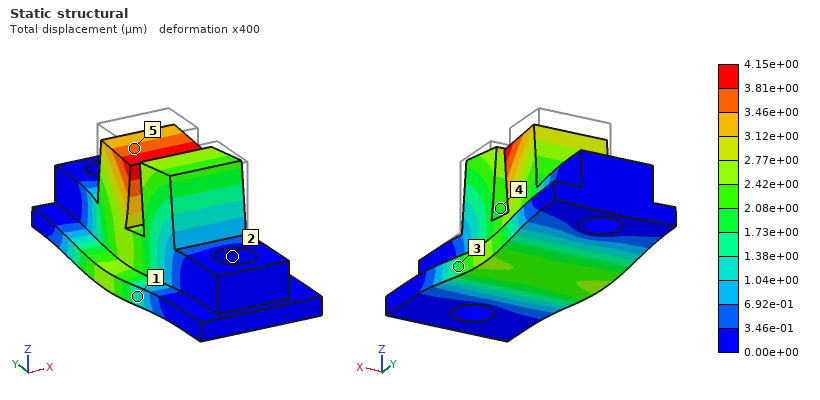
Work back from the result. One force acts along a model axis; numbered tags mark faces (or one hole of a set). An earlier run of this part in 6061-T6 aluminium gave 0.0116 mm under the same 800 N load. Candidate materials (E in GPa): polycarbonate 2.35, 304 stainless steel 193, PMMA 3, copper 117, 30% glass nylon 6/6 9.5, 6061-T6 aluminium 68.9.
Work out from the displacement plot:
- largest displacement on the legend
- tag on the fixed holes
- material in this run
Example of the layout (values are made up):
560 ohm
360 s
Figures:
4.15e+00 µm
2
304 stainless steel
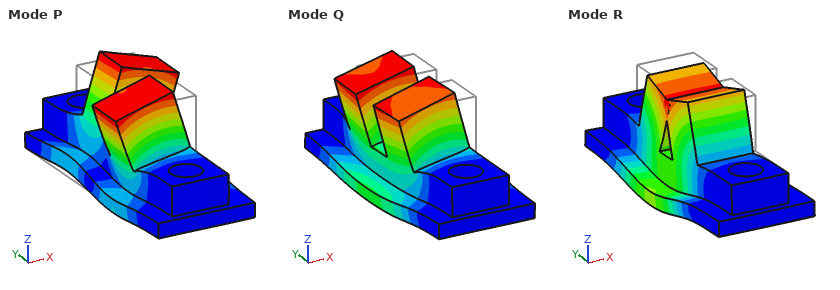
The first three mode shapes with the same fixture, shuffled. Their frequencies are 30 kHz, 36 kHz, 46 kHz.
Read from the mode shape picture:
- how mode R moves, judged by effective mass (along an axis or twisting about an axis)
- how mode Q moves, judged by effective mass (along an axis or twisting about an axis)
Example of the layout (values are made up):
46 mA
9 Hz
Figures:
along Z
along X
